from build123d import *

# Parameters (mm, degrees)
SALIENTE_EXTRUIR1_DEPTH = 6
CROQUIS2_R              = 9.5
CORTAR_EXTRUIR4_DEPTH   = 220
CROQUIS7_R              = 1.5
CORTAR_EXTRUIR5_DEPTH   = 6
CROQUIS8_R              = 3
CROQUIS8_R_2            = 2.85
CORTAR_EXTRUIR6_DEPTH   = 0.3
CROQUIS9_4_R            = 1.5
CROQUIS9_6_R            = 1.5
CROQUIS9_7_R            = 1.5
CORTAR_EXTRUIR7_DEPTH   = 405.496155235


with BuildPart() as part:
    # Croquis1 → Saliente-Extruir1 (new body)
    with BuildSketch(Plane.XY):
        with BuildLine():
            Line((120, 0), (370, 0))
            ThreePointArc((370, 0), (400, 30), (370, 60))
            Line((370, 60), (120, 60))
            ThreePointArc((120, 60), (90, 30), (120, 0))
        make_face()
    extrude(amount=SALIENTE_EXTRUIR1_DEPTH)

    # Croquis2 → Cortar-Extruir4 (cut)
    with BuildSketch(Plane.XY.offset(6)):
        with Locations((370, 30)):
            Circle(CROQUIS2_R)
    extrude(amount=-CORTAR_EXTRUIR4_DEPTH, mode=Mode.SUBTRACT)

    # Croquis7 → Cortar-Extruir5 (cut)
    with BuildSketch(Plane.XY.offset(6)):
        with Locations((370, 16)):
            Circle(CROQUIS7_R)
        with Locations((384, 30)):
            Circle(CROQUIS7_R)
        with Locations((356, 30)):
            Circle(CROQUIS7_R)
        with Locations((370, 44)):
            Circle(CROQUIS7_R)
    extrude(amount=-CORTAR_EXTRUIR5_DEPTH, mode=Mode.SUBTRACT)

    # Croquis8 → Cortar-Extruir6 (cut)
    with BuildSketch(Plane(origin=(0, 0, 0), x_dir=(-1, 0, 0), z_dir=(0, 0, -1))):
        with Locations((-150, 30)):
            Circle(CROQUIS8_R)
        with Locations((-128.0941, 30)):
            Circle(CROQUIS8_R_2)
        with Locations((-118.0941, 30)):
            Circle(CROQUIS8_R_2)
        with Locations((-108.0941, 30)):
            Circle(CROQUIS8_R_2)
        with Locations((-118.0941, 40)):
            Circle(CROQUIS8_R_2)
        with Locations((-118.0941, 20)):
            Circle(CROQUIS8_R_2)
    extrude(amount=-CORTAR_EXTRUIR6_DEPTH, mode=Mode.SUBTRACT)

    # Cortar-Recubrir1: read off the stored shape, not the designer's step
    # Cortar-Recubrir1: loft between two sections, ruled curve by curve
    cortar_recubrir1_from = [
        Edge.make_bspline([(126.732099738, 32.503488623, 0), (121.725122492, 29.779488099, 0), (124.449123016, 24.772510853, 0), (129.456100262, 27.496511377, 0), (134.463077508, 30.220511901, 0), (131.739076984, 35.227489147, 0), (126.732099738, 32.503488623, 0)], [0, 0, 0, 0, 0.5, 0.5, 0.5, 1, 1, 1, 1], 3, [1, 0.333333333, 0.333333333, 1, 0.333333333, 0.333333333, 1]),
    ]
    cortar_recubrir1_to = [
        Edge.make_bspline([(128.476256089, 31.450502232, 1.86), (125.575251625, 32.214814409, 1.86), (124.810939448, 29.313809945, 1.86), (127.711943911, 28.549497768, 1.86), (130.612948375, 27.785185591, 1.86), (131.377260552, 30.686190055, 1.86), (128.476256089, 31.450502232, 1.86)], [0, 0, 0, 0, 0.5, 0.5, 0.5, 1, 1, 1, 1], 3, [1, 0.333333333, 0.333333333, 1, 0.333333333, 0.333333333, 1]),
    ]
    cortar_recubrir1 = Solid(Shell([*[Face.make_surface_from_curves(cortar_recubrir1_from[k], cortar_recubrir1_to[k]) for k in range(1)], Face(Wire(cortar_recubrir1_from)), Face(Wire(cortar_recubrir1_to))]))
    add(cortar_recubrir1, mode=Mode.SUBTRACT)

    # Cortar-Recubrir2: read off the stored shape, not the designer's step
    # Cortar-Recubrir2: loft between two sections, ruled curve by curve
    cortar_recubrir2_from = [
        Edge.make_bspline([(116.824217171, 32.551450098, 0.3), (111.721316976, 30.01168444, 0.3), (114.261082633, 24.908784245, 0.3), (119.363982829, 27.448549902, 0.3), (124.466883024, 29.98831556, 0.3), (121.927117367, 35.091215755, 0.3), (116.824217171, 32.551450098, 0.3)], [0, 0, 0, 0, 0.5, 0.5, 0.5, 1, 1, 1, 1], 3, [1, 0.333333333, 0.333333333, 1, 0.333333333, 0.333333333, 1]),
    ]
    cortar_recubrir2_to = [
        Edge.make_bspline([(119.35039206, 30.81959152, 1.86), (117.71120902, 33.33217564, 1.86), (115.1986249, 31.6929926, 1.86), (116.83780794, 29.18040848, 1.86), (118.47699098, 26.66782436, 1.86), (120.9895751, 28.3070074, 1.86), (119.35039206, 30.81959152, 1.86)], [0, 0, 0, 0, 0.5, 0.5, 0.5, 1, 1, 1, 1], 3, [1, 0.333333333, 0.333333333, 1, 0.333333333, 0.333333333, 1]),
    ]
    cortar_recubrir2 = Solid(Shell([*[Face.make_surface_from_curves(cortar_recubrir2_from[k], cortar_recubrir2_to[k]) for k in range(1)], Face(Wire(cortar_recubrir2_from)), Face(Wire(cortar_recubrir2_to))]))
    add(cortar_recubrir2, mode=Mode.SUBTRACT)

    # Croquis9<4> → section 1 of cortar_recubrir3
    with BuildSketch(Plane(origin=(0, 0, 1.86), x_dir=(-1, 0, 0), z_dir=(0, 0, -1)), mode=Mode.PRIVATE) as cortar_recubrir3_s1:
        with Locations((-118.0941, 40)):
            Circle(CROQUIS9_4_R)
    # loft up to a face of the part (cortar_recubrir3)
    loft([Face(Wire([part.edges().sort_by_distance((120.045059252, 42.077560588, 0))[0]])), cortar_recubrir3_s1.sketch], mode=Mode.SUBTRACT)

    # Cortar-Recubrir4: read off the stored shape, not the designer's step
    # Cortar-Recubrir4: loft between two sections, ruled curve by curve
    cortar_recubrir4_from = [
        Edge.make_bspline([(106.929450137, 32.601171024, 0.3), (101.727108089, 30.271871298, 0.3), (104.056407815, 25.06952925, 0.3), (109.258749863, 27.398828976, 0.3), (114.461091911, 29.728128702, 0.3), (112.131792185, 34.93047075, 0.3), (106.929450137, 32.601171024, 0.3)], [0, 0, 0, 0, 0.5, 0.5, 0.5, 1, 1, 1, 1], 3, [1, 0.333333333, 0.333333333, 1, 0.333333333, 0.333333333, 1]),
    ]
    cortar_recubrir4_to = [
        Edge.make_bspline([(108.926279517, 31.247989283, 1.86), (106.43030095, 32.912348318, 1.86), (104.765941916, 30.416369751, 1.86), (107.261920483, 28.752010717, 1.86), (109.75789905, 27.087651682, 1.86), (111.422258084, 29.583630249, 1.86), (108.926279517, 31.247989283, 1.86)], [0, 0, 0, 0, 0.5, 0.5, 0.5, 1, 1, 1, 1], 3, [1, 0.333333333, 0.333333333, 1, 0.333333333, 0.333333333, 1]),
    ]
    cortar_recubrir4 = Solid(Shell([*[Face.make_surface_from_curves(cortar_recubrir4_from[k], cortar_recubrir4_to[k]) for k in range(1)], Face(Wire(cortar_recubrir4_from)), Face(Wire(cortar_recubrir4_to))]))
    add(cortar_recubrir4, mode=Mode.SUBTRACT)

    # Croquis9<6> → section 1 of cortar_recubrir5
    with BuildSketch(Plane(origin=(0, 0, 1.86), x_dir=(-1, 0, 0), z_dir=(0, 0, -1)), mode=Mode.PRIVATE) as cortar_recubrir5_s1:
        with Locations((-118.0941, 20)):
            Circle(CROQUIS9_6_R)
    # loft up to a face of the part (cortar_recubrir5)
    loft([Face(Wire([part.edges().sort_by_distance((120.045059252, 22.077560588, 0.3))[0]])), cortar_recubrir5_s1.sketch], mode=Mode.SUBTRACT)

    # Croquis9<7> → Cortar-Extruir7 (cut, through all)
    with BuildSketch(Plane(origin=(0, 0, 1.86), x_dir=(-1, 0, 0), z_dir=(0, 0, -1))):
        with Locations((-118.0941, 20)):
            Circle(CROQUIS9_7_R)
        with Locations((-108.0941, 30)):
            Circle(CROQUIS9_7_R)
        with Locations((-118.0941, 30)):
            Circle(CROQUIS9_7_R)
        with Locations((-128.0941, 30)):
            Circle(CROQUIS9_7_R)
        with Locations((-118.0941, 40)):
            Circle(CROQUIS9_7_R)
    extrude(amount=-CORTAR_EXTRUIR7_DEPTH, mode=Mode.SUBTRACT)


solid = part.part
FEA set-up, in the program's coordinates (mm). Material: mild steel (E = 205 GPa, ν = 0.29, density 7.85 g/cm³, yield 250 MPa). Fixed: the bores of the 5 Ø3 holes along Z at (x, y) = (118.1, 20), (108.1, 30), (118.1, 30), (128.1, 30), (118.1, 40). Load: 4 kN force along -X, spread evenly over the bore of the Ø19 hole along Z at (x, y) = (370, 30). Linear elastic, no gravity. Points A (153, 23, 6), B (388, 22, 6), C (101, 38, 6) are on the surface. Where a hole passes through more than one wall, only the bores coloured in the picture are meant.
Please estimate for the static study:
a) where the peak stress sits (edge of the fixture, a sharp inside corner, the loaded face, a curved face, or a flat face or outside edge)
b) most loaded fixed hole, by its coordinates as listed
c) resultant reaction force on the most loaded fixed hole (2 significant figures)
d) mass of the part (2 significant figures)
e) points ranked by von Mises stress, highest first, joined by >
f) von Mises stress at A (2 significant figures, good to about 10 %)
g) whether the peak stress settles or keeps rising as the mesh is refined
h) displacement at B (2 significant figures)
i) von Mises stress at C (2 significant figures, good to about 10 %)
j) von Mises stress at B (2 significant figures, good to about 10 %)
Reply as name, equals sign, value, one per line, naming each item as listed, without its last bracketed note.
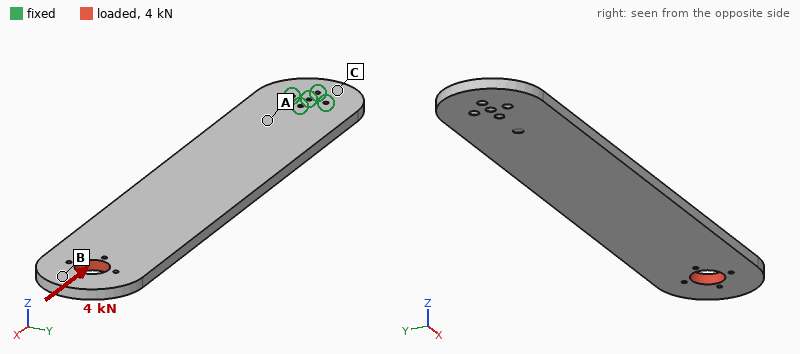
where the peak stress sits = edge of the fixture
most loaded fixed hole, by its coordinates as listed = (128.1, 30)
resultant reaction force on the most loaded fixed hole = 1.3 kN
mass of the part = 820 g
points ranked by von Mises stress, highest first, joined by > = A > B > C
von Mises stress at A = 13 MPa
whether the peak stress settles or keeps rising as the mesh is refined = keeps rising
displacement at B = 19 µm
von Mises stress at C = 4.3 MPa
von Mises stress at B = 8.5 MPa
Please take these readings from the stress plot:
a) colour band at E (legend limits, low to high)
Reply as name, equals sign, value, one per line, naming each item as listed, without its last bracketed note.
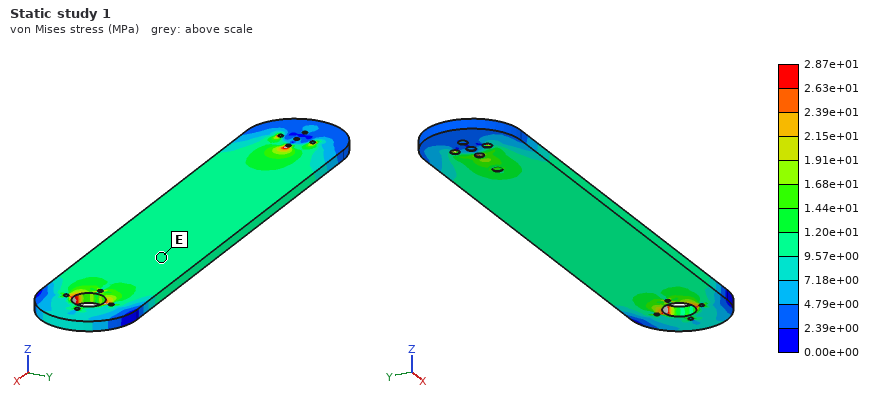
colour band at E = 9.57e+00 to 1.20e+01 MPa
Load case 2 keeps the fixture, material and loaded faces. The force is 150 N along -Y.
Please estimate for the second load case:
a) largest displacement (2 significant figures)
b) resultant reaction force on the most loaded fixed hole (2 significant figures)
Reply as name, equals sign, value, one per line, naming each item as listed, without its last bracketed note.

largest displacement = 60 µm
resultant reaction force on the most loaded fixed hole = 1.0 kN
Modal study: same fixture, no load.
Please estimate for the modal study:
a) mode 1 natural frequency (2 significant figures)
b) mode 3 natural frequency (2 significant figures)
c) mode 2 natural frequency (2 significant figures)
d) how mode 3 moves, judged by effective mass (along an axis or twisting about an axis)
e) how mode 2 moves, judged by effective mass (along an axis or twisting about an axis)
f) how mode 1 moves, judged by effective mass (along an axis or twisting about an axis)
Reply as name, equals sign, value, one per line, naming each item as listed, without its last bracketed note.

mode 1 natural frequency = 70 Hz
mode 3 natural frequency = 540 Hz
mode 2 natural frequency = 430 Hz
how mode 3 moves, judged by effective mass = along Y
how mode 2 moves, judged by effective mass = along Z
how mode 1 moves, judged by effective mass = along Z
